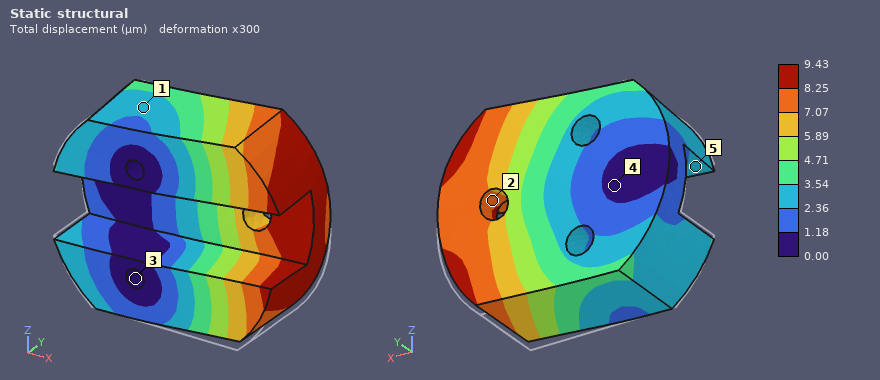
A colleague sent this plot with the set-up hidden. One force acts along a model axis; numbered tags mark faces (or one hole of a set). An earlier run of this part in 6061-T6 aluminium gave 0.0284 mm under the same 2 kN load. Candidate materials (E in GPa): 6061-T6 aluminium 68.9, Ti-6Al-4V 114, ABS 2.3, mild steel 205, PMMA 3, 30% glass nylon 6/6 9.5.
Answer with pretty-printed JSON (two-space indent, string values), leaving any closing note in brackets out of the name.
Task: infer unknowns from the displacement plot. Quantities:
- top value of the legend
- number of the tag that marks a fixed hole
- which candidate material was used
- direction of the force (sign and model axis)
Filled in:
{
  "top value of the legend": "9.43 µm",
  "number of the tag that marks a fixed hole": "3",
  "which candidate material was used": "mild steel",
  "direction of the force": "+Z"
}
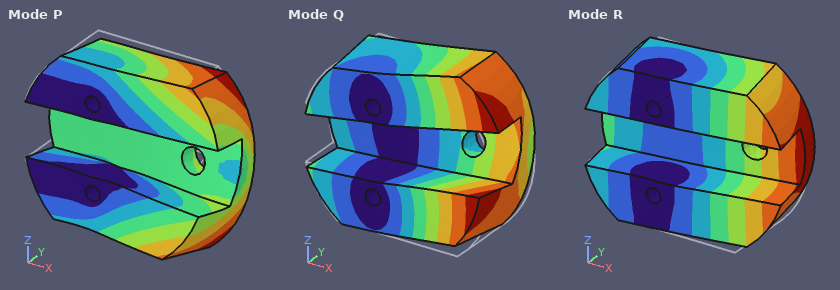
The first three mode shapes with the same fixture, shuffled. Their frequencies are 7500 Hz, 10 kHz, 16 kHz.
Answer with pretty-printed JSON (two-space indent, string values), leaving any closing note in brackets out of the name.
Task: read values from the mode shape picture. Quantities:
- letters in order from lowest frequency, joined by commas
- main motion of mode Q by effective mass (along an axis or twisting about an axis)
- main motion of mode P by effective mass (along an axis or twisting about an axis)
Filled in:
{
  "letters in order from lowest frequency, joined by commas": "R, Q, P",
  "main motion of mode Q by effective mass": "along Z",
  "main motion of mode P by effective mass": "along Z"
}
